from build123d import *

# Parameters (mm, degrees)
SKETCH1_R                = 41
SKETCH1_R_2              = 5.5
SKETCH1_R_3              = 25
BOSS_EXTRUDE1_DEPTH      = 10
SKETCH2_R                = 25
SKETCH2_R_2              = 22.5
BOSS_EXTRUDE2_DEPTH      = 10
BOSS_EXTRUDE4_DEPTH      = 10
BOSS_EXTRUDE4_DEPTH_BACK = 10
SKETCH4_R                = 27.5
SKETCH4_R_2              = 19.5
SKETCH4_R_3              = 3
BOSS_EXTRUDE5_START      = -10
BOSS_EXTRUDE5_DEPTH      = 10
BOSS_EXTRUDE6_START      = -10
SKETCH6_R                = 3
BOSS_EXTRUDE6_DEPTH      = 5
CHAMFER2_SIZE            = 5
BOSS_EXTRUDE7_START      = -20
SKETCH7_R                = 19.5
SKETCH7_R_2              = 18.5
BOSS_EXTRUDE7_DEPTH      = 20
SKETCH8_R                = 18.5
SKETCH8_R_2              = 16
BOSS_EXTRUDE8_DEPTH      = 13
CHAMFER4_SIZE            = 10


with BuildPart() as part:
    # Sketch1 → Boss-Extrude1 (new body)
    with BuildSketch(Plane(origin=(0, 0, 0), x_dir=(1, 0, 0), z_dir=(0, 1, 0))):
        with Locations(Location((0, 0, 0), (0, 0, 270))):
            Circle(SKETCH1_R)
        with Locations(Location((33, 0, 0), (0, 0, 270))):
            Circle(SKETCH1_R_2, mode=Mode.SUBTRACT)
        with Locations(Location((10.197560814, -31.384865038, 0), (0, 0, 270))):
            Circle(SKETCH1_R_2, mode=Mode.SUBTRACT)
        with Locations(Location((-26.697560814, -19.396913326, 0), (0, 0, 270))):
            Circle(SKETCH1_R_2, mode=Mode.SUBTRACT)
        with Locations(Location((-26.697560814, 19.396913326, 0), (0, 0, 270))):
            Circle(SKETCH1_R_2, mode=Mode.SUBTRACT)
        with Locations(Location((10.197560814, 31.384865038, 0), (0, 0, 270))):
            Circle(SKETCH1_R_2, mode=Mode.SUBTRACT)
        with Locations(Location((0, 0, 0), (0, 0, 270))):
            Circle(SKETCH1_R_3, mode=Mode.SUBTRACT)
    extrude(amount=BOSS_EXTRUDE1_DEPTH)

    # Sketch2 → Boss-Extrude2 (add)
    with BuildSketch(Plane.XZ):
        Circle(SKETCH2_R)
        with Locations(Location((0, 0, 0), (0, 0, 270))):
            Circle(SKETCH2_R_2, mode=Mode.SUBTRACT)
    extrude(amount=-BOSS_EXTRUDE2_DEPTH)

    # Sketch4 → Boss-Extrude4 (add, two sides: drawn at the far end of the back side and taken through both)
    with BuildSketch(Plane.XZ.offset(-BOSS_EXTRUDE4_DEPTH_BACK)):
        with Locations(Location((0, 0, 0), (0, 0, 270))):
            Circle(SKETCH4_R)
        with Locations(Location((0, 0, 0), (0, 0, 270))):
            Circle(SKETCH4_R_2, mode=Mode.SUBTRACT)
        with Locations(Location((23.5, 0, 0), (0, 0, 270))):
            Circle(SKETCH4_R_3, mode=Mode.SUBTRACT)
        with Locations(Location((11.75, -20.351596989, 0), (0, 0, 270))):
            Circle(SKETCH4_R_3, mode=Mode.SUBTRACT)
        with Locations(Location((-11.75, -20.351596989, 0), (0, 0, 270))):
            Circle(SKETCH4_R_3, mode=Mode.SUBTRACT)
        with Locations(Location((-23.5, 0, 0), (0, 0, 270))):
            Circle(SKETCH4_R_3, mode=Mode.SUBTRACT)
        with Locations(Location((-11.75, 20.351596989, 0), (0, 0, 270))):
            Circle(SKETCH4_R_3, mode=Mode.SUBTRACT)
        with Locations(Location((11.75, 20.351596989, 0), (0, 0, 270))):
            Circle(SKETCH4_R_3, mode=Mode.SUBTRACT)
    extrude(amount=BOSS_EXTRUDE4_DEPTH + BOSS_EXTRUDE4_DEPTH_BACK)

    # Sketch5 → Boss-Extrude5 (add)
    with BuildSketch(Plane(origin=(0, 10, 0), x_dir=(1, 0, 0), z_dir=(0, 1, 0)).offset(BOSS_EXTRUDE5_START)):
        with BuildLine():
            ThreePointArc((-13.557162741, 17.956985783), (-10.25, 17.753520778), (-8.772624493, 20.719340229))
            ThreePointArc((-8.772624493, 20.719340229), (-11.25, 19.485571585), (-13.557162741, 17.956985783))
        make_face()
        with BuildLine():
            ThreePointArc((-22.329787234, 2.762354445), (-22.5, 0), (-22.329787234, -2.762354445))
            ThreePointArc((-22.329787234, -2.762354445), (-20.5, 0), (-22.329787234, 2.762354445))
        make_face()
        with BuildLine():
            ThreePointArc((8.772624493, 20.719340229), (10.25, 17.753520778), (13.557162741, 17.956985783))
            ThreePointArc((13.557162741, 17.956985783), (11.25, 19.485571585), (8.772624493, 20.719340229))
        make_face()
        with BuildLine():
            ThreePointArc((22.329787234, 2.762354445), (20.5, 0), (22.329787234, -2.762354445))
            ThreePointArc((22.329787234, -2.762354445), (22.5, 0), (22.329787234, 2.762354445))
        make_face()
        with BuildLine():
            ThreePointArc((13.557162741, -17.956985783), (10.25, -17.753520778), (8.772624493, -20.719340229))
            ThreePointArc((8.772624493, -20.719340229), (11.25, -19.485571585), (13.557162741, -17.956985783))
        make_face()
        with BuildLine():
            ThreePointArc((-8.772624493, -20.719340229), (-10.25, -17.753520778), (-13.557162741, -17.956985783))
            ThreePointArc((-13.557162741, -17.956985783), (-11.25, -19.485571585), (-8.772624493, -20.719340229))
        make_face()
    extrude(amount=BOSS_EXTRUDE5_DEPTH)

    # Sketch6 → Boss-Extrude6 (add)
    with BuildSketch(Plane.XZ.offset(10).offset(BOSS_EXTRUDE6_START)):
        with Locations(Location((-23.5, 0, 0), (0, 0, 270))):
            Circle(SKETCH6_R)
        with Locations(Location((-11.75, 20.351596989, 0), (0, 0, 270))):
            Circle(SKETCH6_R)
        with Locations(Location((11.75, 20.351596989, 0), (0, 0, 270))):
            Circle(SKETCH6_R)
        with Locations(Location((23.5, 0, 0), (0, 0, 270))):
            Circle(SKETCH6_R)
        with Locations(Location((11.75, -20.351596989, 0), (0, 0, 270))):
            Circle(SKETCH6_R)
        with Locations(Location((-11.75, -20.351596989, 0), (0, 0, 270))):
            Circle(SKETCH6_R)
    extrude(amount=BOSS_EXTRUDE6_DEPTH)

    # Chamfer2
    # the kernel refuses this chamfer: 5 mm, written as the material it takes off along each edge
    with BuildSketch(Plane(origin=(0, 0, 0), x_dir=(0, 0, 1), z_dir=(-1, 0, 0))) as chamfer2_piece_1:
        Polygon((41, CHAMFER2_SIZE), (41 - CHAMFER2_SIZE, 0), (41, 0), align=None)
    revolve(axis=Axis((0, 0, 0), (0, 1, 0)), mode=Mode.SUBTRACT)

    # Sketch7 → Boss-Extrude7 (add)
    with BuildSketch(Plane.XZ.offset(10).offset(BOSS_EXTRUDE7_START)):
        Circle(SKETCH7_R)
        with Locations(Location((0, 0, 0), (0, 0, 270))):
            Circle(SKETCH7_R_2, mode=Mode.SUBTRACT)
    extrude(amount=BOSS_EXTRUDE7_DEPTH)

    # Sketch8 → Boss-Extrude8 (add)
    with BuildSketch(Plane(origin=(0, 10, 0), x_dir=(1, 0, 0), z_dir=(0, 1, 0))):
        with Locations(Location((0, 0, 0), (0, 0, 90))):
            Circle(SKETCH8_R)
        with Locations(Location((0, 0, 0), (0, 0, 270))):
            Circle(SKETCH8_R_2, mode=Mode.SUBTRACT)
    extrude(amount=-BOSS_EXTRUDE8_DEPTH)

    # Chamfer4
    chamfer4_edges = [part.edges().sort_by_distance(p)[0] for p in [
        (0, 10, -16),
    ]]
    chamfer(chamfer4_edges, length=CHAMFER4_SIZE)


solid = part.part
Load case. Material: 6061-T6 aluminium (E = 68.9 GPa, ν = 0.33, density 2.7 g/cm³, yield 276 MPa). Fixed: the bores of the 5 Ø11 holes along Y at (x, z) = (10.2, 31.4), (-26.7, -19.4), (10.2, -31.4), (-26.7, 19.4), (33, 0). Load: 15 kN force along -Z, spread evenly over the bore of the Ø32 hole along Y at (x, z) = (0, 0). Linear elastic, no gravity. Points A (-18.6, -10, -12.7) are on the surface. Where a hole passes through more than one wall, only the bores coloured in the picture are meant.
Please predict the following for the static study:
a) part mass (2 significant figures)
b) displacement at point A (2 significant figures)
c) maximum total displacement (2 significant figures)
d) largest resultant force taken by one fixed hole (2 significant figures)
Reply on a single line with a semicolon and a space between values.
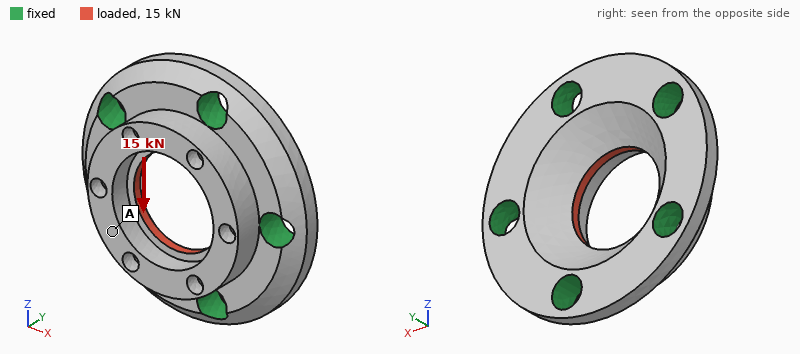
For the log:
120 g; 5.3 µm; 13 µm; 3.6 kN
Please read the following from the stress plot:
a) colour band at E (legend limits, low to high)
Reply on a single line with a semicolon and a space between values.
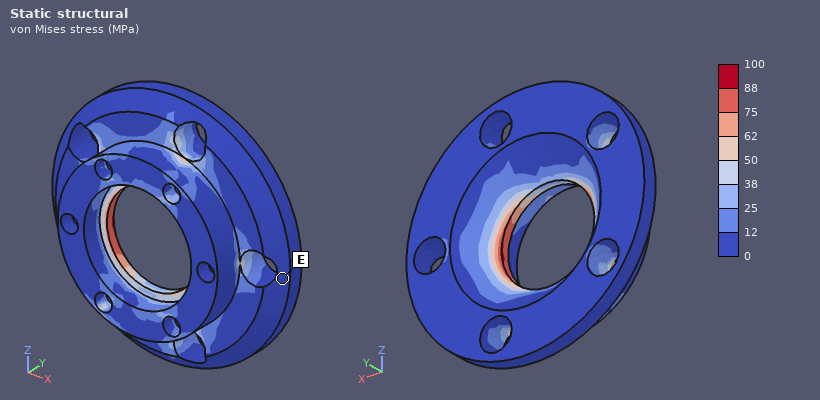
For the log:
0 to 12 MPa
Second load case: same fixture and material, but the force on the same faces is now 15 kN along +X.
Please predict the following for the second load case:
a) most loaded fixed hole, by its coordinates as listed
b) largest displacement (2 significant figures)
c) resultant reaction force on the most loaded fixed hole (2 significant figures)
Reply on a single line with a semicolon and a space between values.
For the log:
(33, 0); 13 µm; 3.7 kN
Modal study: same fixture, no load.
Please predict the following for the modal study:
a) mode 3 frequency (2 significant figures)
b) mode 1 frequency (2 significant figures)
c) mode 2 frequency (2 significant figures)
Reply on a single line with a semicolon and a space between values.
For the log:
30 kHz; 29 kHz; 30 kHz
